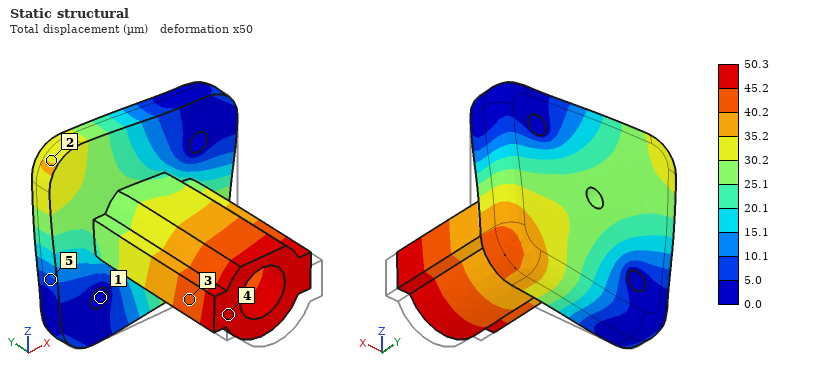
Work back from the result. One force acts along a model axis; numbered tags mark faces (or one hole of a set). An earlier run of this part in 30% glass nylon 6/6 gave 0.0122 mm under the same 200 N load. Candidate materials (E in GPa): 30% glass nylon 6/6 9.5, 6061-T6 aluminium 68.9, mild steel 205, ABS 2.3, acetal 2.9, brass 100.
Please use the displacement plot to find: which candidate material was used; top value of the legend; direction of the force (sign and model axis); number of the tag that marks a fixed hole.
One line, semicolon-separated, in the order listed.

ABS; 50.3 µm; +Y; 1
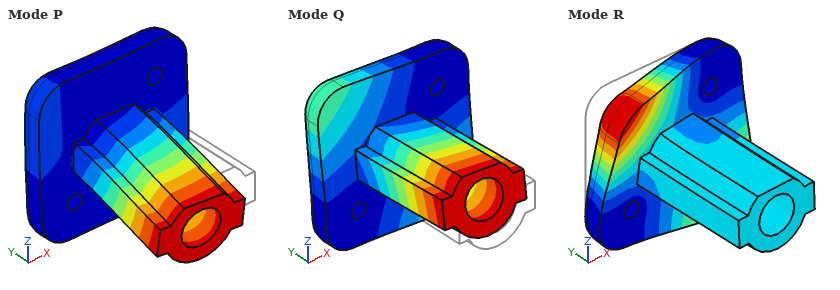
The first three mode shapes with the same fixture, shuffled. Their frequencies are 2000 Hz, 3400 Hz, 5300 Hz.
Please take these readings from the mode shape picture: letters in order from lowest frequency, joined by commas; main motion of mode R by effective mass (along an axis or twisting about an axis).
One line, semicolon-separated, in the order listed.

Q, P, R; along Y
